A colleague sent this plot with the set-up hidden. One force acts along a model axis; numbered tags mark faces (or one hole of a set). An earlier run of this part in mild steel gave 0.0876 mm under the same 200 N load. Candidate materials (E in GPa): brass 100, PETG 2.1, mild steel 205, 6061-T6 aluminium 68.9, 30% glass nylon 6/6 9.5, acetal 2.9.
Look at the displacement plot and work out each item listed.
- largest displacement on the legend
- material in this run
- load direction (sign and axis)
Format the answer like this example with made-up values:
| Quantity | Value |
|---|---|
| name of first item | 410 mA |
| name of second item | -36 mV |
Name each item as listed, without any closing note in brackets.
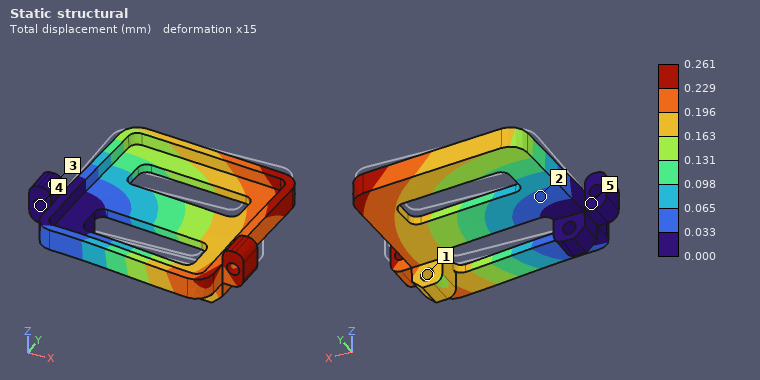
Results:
| Quantity | Value |
|---|---|
| largest displacement on the legend | 0.261 mm |
| material in this run | 6061-T6 aluminium |
| load direction | -Y |
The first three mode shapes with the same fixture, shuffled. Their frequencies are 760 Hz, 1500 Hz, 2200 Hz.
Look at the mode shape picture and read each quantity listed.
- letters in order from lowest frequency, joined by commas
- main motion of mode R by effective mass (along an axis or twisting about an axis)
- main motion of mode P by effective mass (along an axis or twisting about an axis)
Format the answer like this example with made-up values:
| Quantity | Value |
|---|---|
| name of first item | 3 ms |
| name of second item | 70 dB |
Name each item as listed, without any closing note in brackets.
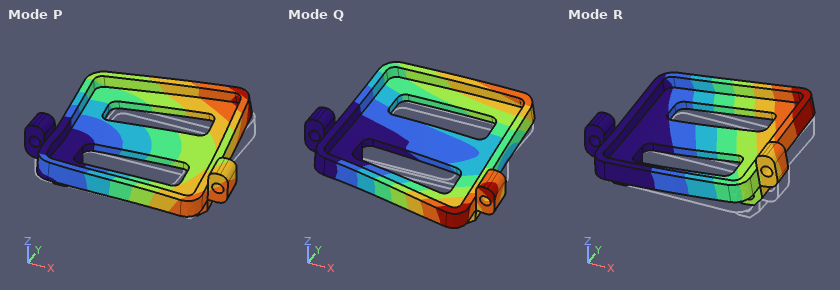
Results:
| Quantity | Value |
|---|---|
| letters in order from lowest frequency, joined by commas | R, Q, P |
| main motion of mode R by effective mass | along Z |
| main motion of mode P by effective mass | along Y |
